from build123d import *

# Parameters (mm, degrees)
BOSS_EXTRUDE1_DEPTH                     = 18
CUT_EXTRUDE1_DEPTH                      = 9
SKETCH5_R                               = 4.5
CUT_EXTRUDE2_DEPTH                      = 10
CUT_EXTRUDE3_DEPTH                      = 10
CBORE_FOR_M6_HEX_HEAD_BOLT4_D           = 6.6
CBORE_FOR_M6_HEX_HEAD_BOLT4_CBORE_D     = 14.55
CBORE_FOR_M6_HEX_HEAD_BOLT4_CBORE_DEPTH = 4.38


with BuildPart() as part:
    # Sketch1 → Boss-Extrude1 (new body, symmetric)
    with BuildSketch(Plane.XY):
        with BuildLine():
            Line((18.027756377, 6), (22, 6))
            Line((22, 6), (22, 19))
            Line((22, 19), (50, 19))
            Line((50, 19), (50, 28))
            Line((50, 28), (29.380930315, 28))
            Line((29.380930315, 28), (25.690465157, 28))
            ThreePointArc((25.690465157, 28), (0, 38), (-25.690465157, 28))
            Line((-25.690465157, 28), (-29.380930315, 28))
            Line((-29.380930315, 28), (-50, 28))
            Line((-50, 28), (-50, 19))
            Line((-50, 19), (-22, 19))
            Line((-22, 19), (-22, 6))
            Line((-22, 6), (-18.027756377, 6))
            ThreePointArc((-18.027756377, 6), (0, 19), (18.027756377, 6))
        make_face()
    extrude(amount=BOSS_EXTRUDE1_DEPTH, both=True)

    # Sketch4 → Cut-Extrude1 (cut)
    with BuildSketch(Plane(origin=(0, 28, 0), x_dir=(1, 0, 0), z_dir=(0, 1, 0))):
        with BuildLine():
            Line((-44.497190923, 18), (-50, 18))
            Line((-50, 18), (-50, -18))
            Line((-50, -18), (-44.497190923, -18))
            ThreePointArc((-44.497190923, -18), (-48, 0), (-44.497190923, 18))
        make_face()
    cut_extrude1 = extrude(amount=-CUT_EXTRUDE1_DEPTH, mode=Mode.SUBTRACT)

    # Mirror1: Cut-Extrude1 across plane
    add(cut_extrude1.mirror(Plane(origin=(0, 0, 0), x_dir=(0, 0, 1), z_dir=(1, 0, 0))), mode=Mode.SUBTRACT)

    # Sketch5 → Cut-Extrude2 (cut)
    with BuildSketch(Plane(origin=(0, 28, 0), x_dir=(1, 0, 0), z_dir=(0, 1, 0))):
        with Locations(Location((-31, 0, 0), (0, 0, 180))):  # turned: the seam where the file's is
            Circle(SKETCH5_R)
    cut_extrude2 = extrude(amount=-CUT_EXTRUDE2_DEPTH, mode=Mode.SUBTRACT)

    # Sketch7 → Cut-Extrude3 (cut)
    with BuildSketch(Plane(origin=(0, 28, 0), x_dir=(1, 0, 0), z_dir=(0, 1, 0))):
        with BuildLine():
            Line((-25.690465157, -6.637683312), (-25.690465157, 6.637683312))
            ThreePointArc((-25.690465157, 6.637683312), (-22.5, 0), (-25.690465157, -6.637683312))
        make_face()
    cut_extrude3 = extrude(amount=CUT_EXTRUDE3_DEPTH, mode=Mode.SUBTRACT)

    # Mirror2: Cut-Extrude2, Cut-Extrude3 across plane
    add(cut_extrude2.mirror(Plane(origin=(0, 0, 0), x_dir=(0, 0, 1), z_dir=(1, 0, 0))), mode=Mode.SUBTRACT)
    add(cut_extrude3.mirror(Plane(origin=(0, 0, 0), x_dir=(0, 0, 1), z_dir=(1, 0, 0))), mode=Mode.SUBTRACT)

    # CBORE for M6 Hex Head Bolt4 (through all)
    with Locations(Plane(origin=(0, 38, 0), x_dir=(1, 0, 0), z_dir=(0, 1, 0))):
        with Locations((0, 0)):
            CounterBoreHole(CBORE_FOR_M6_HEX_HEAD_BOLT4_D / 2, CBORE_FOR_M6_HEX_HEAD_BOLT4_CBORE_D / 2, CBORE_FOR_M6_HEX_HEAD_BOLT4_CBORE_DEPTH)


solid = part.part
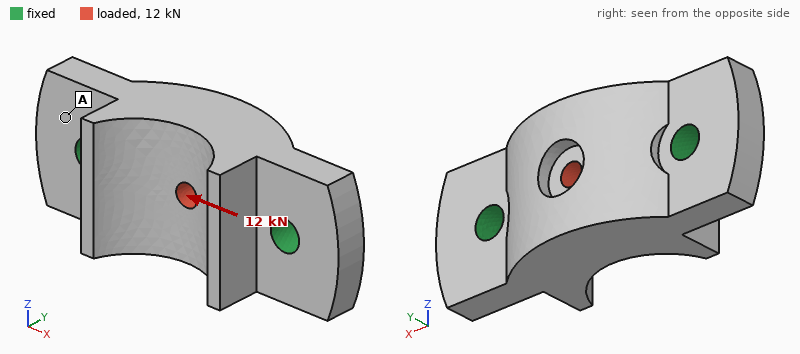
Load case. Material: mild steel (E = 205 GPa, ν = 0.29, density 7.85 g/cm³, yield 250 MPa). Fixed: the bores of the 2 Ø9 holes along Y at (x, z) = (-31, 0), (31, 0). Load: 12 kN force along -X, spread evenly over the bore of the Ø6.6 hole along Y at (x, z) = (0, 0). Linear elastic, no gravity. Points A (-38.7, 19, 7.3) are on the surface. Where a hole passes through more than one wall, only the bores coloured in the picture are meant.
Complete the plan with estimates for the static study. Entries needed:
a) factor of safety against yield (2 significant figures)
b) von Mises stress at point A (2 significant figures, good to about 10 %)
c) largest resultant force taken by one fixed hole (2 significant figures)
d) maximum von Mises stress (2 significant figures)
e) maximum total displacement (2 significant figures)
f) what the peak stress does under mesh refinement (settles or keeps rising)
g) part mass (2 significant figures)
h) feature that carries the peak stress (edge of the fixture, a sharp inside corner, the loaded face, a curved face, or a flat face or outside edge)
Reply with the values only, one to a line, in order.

3.6
9.0 MPa
6.0 kN
68 MPa
3.4 µm
settles
380 g
the loaded face
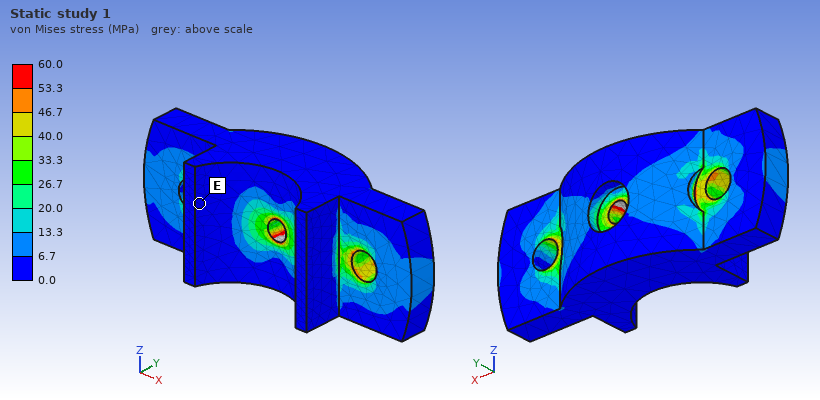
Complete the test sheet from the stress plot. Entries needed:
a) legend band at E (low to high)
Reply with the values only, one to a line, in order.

0.0 to 6.7 MPa
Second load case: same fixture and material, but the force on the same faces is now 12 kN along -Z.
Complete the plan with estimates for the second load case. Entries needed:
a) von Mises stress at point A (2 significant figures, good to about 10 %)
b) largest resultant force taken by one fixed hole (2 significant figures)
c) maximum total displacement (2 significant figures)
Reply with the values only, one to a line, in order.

12 MPa
6.0 kN
12 µm
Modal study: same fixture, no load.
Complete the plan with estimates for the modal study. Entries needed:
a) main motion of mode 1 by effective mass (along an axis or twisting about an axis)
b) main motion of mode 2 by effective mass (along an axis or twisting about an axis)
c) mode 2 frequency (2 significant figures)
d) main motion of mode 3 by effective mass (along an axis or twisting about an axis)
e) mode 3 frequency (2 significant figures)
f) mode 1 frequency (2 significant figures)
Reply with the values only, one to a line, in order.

twisting about X
along Y
11 kHz
along Z
15 kHz
9100 Hz
